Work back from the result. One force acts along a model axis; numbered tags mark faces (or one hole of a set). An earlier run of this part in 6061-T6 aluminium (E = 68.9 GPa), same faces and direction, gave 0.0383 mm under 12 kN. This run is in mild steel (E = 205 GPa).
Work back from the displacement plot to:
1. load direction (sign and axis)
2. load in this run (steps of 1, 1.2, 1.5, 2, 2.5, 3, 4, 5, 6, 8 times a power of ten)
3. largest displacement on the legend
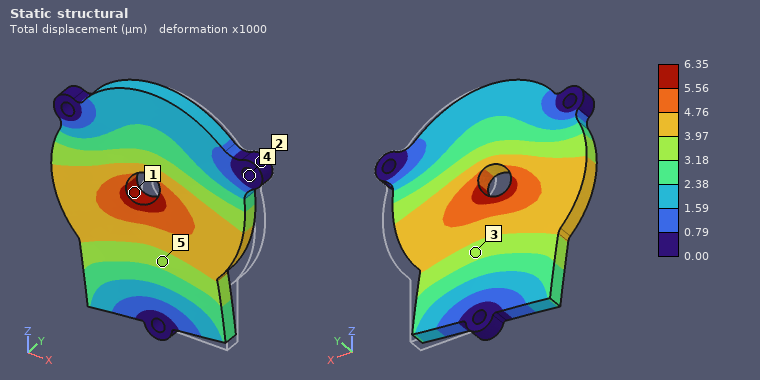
-X
6 kN
6.35 µm
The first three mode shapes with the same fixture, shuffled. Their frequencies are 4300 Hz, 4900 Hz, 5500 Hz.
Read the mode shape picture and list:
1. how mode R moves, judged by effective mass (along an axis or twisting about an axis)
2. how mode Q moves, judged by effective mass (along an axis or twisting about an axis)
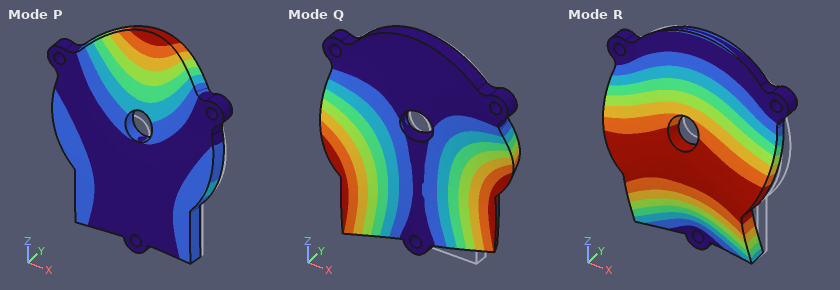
along Y
twisting about Z
